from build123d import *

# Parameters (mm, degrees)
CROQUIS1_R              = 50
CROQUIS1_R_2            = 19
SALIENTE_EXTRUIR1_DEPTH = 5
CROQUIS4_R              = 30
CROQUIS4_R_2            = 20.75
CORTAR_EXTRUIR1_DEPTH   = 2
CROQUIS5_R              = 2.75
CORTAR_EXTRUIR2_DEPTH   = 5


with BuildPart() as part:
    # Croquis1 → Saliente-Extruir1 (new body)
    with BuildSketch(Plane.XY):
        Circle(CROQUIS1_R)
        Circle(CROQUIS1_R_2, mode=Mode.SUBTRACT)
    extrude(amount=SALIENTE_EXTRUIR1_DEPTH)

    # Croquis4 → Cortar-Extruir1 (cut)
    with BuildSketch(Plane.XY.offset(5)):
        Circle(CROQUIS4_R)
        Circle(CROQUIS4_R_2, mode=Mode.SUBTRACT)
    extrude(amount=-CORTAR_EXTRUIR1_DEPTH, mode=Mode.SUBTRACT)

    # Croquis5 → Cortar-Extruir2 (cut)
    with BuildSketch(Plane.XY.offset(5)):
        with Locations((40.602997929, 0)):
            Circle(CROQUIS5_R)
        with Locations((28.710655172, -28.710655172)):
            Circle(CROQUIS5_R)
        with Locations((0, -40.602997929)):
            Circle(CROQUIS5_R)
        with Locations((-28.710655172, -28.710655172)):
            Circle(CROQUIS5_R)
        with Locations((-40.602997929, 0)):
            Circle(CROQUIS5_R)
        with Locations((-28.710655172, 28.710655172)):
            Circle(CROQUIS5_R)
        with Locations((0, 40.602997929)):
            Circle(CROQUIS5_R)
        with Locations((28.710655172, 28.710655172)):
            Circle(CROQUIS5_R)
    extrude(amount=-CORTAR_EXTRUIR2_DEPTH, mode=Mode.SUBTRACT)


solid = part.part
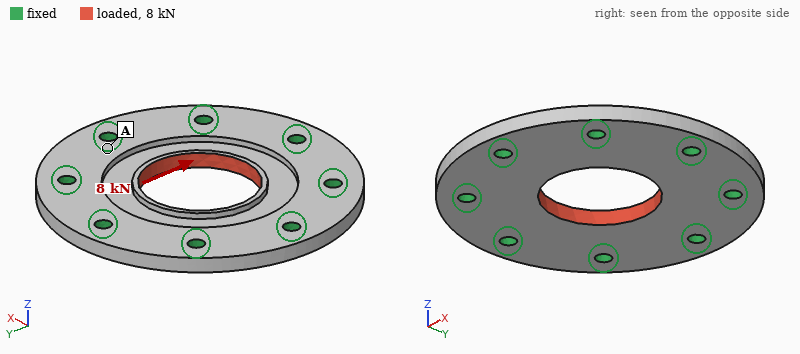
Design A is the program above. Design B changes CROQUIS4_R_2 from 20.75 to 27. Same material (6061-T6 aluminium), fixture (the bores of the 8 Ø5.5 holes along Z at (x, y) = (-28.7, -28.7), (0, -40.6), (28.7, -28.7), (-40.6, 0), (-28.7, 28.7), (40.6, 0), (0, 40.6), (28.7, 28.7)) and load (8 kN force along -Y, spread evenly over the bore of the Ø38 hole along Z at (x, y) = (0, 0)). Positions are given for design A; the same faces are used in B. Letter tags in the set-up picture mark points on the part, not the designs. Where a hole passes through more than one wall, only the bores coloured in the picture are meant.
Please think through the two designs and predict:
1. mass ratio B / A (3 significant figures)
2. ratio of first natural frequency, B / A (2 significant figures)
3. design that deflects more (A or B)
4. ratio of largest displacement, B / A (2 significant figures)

1.06
0.93
A
0.61
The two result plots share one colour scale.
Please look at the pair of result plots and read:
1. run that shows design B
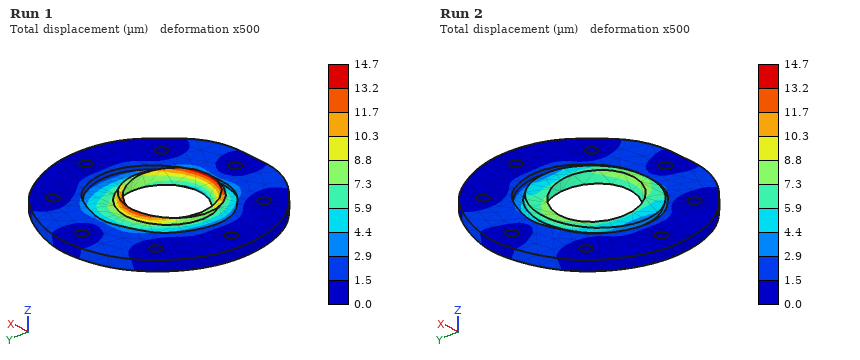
Run 2
